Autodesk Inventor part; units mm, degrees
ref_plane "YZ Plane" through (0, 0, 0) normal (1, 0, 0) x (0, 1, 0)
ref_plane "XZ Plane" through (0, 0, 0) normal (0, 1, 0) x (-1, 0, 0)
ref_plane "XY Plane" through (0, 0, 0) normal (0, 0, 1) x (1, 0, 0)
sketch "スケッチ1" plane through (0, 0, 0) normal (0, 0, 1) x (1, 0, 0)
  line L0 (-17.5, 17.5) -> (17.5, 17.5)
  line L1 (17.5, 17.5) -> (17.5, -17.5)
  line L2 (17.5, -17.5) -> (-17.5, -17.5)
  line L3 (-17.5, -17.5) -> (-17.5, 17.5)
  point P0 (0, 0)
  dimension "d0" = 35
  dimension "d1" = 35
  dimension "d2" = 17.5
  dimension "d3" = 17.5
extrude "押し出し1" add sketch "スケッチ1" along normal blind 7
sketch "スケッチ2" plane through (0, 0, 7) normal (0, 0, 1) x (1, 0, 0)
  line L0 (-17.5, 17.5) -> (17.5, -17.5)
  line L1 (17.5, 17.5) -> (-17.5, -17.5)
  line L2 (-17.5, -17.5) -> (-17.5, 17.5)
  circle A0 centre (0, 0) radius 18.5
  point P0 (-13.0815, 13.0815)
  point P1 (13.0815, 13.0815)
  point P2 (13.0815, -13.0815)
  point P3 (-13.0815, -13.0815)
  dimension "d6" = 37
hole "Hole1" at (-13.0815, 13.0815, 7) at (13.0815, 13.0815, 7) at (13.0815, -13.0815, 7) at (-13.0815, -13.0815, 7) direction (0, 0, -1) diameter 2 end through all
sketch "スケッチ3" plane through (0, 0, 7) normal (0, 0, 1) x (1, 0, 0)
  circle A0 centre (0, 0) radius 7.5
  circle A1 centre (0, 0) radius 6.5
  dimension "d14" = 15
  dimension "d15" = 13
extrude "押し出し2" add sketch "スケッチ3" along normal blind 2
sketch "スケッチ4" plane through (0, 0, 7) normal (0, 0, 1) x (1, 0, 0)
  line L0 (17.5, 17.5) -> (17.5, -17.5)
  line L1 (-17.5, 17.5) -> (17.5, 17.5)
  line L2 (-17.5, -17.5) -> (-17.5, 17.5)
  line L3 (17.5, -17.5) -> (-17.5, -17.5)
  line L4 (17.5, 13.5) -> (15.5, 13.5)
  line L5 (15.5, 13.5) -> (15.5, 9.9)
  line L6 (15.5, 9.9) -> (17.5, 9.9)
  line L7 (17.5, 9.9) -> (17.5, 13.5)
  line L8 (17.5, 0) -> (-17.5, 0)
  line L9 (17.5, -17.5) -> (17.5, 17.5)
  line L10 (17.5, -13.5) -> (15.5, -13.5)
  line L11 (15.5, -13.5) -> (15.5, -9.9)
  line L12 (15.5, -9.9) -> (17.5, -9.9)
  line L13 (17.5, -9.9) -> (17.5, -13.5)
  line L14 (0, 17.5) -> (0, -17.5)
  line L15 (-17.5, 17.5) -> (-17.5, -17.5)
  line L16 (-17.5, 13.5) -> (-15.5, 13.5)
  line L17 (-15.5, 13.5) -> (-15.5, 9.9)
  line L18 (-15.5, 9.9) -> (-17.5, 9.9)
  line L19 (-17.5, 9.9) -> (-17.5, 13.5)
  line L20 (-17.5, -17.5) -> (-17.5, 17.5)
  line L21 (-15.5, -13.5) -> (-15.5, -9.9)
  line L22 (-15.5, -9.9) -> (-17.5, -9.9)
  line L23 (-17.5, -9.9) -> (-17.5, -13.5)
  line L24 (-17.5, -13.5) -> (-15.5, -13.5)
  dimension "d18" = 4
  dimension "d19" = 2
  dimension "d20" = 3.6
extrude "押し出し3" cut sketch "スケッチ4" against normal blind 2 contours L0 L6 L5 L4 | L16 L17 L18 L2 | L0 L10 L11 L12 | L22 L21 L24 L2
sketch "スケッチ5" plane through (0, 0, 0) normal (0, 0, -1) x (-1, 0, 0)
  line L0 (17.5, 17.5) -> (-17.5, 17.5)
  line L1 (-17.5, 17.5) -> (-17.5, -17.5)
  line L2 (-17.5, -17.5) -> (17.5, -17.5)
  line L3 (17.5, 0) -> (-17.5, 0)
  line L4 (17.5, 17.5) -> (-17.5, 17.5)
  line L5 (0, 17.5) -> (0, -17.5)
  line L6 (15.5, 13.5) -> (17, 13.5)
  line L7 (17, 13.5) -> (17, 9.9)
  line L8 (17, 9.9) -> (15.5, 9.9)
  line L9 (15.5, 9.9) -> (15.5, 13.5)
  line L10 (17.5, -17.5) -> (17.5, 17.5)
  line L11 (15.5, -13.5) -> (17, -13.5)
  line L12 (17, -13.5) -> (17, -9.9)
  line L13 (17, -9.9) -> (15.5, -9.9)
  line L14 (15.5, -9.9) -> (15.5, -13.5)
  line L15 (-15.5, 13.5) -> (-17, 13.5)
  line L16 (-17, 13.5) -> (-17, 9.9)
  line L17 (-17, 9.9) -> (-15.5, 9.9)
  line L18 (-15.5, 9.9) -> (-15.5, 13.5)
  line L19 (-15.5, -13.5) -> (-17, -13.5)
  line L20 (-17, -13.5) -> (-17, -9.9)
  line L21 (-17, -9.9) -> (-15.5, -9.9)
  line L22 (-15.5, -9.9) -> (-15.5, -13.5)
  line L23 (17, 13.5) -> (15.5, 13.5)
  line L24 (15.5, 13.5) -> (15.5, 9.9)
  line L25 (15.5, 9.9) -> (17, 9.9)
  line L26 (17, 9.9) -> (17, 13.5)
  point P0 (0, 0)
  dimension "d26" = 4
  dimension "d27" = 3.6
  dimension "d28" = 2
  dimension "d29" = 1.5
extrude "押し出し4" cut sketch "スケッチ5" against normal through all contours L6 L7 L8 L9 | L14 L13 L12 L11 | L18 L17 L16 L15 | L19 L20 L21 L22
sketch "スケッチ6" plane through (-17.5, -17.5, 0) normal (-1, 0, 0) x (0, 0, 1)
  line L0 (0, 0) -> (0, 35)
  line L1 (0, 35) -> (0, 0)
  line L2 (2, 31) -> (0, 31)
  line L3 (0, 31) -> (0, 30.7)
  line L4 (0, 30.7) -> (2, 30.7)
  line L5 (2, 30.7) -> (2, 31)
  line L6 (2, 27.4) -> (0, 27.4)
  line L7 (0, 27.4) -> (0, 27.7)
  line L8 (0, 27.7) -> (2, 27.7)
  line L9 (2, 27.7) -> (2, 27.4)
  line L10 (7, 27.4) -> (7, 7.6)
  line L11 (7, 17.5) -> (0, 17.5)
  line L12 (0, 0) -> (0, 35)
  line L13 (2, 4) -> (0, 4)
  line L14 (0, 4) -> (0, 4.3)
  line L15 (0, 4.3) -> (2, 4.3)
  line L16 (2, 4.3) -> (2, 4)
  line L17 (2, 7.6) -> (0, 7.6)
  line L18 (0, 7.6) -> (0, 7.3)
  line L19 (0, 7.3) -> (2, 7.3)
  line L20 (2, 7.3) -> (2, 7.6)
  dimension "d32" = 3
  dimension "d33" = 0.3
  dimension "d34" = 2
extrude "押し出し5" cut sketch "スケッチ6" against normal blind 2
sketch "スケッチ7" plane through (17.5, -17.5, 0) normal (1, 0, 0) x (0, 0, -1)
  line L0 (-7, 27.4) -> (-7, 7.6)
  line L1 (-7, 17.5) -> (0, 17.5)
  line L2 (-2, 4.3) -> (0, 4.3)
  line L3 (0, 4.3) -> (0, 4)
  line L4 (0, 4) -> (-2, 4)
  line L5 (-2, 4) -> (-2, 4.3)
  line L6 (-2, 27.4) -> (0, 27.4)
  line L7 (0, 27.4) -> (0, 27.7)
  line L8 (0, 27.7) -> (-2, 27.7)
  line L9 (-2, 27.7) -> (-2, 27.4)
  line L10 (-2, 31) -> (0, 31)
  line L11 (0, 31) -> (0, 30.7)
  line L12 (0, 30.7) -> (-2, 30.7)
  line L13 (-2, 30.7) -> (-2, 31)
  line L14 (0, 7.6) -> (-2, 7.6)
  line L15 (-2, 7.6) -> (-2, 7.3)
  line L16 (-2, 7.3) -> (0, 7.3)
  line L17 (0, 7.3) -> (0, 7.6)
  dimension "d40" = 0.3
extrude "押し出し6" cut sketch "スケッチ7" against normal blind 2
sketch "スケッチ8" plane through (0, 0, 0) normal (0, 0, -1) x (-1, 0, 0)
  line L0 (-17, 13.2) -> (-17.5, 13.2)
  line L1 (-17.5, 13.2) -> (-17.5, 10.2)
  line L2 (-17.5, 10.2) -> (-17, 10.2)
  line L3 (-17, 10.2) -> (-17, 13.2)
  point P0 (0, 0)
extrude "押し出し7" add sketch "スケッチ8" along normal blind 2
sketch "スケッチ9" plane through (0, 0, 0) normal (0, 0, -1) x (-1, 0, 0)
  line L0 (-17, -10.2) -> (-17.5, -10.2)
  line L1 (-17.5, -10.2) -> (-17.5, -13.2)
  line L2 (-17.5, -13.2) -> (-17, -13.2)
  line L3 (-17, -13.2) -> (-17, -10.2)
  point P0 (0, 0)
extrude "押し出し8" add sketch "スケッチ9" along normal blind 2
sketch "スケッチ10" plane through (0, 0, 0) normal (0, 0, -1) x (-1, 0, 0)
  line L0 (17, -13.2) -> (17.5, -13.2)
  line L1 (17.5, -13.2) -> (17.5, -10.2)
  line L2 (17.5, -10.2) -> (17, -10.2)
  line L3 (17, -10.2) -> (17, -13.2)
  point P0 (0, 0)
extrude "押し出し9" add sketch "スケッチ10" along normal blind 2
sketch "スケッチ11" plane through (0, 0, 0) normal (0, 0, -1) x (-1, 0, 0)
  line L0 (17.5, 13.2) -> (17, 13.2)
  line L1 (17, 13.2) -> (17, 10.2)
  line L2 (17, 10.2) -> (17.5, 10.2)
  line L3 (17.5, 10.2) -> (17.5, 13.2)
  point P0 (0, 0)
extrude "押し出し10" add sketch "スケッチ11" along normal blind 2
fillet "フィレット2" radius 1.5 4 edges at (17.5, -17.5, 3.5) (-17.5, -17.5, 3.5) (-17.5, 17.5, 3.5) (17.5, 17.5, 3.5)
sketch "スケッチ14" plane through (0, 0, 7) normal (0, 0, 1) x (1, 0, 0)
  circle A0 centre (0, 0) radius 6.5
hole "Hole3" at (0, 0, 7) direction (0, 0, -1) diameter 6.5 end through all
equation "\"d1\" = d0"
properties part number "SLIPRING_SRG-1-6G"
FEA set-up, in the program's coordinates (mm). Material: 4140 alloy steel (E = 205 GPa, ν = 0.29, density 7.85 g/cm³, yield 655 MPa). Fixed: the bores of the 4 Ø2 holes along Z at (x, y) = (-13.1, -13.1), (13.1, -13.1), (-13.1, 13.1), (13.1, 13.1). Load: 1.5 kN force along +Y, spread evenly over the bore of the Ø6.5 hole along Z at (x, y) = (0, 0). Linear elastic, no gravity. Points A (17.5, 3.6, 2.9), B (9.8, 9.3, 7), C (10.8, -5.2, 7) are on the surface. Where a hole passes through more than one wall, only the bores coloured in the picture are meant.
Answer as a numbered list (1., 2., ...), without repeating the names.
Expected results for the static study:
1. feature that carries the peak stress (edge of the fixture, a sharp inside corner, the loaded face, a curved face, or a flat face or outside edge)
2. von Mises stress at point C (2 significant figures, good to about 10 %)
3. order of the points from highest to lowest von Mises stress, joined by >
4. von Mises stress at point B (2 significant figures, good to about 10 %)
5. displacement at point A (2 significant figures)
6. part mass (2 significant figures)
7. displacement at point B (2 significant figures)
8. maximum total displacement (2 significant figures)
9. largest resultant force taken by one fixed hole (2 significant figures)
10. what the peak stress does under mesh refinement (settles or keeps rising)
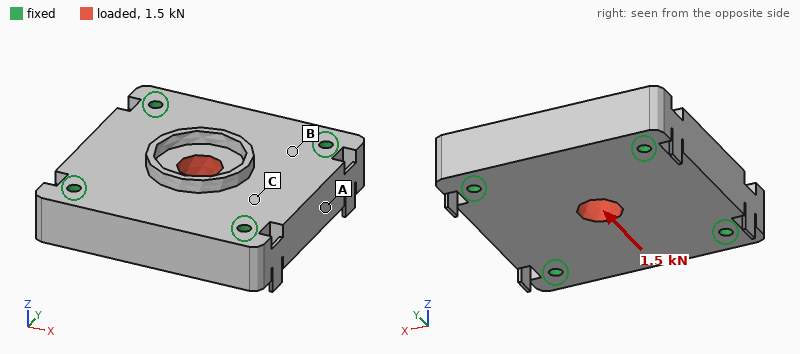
1. edge of the fixture
2. 5.1 MPa
3. B > C > A
4. 8.0 MPa
5. 0.14 µm
6. 64 g
7. 0.24 µm
8. 0.79 µm
9. 410 N
10. keeps rising
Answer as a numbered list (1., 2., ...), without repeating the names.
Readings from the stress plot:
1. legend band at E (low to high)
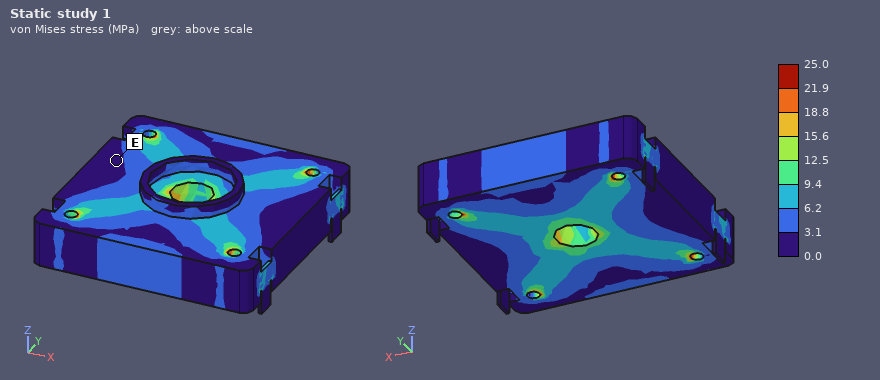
1. 0.0 to 3.1 MPa
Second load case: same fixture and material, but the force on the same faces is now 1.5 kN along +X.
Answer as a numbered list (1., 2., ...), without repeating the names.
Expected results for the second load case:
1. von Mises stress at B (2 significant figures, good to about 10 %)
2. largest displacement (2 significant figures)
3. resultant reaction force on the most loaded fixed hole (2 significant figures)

1. 8.0 MPa
2. 0.79 µm
3. 410 N
